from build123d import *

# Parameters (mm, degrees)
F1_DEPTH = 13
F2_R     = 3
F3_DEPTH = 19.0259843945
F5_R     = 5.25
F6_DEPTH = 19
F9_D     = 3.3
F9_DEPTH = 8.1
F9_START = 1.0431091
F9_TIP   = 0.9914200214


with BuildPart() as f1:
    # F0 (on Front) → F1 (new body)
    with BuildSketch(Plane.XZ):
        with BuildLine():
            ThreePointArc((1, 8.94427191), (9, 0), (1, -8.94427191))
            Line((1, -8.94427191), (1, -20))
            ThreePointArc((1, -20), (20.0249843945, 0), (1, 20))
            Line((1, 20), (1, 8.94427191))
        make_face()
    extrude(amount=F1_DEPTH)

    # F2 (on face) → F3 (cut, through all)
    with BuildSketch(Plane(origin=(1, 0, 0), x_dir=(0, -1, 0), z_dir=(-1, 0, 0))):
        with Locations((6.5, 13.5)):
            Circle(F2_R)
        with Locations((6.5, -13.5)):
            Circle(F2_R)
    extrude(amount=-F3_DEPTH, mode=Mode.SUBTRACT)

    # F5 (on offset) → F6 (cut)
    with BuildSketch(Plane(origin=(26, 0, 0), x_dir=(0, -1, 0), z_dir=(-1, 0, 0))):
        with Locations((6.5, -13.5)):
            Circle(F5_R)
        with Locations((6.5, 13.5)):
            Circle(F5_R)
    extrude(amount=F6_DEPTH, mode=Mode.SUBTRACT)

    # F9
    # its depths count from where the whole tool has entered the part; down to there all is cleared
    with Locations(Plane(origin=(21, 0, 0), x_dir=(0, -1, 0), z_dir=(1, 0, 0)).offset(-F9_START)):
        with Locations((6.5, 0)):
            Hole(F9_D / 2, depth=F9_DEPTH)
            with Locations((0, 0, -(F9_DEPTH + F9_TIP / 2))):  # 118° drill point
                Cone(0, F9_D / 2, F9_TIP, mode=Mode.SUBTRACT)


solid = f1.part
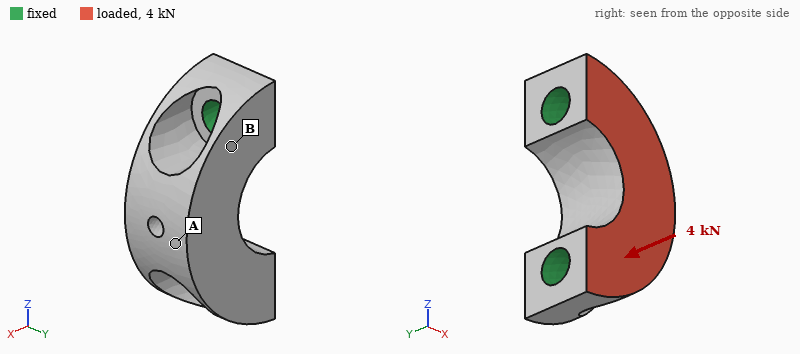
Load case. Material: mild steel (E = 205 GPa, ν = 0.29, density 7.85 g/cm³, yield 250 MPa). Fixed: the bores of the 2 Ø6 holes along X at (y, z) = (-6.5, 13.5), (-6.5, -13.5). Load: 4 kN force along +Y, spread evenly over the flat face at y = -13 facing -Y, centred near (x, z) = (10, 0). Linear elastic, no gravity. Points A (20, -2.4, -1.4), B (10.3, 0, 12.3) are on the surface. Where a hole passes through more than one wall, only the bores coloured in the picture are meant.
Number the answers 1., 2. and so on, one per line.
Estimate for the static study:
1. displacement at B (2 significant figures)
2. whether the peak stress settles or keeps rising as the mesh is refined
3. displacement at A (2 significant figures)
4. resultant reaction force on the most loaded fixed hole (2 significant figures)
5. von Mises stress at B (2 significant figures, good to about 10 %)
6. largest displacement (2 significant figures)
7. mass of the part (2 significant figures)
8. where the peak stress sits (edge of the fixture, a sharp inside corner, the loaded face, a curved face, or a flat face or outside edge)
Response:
1. 5.2 µm
2. keeps rising
3. 13 µm
4. 2.0 kN
5. 41 MPa
6. 14 µm
7. 36 g
8. edge of the fixture
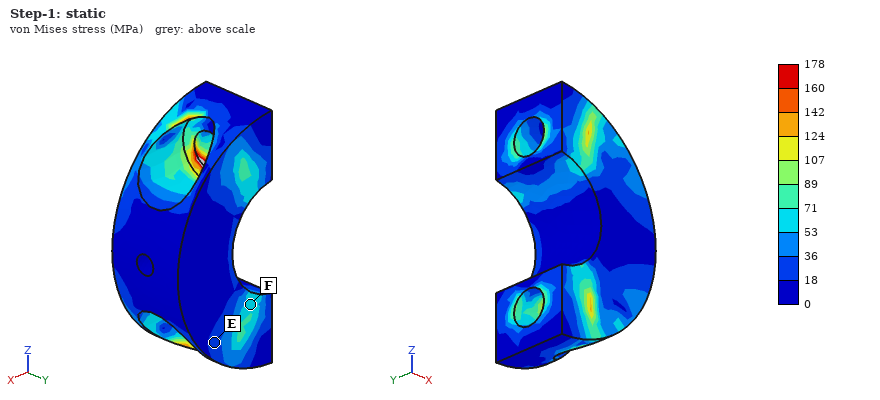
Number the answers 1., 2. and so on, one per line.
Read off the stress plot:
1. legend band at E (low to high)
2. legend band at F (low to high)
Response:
1. 18 to 36 MPa
2. 53 to 71 MPa
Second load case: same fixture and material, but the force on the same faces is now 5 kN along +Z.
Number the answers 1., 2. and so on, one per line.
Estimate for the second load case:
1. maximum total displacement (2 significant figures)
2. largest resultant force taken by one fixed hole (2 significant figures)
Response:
1. 8.5 µm
2. 2.8 kN
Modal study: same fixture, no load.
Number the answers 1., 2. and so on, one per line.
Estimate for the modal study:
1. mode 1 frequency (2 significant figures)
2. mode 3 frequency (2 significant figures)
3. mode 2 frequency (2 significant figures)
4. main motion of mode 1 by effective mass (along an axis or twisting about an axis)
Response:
1. 17 kHz
2. 36 kHz
3. 36 kHz
4. along Y
